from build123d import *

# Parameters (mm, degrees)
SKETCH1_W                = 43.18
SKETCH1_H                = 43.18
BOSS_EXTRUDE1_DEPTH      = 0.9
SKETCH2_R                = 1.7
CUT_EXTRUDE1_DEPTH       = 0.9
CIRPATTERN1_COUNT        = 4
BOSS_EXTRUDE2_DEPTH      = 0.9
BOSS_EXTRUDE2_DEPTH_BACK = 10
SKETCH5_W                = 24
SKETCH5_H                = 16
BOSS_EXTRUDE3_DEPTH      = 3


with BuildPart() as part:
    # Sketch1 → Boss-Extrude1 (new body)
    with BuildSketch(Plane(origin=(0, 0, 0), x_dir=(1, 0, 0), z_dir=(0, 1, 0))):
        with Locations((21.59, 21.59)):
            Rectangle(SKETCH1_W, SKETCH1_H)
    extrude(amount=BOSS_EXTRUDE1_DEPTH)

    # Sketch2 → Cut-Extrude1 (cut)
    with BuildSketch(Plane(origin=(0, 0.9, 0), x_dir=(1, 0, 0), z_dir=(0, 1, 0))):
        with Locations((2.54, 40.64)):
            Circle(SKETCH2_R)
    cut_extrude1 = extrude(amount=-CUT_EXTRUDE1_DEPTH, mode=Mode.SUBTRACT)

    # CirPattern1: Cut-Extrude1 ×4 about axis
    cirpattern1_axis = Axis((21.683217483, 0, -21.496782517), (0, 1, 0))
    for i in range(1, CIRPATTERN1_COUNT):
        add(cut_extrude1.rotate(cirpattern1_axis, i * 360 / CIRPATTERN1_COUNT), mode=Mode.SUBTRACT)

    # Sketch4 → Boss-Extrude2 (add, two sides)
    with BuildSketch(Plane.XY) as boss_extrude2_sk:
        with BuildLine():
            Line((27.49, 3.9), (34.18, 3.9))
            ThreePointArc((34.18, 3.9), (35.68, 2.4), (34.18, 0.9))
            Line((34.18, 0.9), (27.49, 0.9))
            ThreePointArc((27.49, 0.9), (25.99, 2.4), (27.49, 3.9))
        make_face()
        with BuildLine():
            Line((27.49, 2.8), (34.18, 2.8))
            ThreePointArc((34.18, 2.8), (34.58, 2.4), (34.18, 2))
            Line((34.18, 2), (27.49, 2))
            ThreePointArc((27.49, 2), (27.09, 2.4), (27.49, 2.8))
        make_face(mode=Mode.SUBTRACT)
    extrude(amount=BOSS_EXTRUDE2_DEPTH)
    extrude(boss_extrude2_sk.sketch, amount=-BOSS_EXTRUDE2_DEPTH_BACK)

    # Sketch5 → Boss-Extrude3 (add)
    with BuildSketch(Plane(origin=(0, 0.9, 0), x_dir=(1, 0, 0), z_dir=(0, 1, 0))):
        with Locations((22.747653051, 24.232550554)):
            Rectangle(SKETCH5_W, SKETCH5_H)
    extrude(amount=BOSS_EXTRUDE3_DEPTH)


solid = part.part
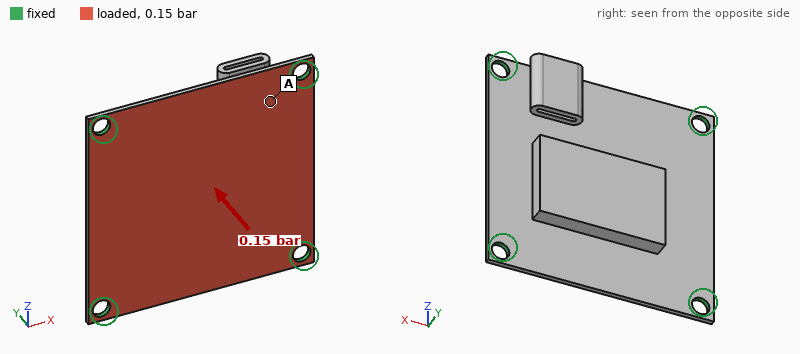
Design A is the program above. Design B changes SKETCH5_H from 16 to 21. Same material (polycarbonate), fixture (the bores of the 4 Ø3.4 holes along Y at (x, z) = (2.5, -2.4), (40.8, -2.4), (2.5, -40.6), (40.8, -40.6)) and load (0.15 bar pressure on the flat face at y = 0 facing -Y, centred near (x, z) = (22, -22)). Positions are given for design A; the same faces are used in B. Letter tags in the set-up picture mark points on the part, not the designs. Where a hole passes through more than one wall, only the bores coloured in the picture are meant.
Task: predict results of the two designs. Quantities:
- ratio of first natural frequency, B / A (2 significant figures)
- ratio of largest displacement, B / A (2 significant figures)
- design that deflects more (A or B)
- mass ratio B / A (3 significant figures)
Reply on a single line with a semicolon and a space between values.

1.1; 0.78; A; 1.12
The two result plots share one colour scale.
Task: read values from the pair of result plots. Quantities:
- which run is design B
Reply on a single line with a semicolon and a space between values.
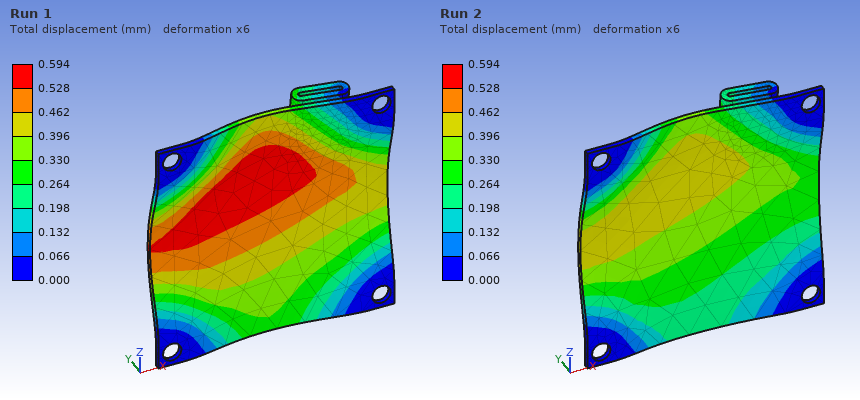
Run 2
